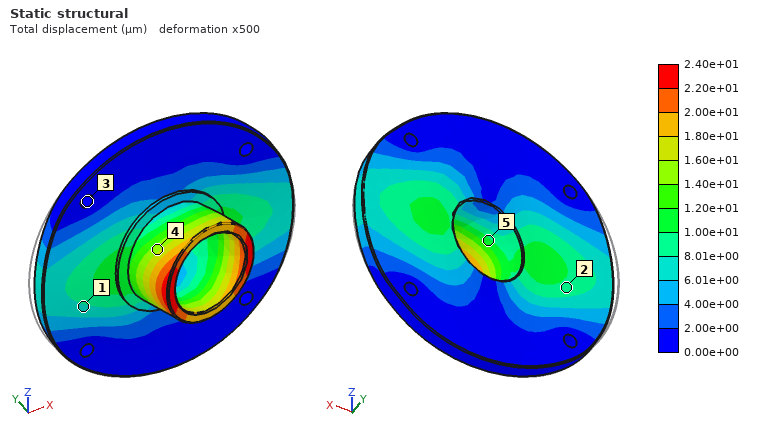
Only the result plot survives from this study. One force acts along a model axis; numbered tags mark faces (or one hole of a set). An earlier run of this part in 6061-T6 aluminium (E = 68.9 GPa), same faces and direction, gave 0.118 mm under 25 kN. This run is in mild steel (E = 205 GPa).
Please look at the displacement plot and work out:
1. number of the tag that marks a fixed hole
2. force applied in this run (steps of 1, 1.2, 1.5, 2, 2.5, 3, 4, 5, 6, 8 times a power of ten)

3
15 kN
